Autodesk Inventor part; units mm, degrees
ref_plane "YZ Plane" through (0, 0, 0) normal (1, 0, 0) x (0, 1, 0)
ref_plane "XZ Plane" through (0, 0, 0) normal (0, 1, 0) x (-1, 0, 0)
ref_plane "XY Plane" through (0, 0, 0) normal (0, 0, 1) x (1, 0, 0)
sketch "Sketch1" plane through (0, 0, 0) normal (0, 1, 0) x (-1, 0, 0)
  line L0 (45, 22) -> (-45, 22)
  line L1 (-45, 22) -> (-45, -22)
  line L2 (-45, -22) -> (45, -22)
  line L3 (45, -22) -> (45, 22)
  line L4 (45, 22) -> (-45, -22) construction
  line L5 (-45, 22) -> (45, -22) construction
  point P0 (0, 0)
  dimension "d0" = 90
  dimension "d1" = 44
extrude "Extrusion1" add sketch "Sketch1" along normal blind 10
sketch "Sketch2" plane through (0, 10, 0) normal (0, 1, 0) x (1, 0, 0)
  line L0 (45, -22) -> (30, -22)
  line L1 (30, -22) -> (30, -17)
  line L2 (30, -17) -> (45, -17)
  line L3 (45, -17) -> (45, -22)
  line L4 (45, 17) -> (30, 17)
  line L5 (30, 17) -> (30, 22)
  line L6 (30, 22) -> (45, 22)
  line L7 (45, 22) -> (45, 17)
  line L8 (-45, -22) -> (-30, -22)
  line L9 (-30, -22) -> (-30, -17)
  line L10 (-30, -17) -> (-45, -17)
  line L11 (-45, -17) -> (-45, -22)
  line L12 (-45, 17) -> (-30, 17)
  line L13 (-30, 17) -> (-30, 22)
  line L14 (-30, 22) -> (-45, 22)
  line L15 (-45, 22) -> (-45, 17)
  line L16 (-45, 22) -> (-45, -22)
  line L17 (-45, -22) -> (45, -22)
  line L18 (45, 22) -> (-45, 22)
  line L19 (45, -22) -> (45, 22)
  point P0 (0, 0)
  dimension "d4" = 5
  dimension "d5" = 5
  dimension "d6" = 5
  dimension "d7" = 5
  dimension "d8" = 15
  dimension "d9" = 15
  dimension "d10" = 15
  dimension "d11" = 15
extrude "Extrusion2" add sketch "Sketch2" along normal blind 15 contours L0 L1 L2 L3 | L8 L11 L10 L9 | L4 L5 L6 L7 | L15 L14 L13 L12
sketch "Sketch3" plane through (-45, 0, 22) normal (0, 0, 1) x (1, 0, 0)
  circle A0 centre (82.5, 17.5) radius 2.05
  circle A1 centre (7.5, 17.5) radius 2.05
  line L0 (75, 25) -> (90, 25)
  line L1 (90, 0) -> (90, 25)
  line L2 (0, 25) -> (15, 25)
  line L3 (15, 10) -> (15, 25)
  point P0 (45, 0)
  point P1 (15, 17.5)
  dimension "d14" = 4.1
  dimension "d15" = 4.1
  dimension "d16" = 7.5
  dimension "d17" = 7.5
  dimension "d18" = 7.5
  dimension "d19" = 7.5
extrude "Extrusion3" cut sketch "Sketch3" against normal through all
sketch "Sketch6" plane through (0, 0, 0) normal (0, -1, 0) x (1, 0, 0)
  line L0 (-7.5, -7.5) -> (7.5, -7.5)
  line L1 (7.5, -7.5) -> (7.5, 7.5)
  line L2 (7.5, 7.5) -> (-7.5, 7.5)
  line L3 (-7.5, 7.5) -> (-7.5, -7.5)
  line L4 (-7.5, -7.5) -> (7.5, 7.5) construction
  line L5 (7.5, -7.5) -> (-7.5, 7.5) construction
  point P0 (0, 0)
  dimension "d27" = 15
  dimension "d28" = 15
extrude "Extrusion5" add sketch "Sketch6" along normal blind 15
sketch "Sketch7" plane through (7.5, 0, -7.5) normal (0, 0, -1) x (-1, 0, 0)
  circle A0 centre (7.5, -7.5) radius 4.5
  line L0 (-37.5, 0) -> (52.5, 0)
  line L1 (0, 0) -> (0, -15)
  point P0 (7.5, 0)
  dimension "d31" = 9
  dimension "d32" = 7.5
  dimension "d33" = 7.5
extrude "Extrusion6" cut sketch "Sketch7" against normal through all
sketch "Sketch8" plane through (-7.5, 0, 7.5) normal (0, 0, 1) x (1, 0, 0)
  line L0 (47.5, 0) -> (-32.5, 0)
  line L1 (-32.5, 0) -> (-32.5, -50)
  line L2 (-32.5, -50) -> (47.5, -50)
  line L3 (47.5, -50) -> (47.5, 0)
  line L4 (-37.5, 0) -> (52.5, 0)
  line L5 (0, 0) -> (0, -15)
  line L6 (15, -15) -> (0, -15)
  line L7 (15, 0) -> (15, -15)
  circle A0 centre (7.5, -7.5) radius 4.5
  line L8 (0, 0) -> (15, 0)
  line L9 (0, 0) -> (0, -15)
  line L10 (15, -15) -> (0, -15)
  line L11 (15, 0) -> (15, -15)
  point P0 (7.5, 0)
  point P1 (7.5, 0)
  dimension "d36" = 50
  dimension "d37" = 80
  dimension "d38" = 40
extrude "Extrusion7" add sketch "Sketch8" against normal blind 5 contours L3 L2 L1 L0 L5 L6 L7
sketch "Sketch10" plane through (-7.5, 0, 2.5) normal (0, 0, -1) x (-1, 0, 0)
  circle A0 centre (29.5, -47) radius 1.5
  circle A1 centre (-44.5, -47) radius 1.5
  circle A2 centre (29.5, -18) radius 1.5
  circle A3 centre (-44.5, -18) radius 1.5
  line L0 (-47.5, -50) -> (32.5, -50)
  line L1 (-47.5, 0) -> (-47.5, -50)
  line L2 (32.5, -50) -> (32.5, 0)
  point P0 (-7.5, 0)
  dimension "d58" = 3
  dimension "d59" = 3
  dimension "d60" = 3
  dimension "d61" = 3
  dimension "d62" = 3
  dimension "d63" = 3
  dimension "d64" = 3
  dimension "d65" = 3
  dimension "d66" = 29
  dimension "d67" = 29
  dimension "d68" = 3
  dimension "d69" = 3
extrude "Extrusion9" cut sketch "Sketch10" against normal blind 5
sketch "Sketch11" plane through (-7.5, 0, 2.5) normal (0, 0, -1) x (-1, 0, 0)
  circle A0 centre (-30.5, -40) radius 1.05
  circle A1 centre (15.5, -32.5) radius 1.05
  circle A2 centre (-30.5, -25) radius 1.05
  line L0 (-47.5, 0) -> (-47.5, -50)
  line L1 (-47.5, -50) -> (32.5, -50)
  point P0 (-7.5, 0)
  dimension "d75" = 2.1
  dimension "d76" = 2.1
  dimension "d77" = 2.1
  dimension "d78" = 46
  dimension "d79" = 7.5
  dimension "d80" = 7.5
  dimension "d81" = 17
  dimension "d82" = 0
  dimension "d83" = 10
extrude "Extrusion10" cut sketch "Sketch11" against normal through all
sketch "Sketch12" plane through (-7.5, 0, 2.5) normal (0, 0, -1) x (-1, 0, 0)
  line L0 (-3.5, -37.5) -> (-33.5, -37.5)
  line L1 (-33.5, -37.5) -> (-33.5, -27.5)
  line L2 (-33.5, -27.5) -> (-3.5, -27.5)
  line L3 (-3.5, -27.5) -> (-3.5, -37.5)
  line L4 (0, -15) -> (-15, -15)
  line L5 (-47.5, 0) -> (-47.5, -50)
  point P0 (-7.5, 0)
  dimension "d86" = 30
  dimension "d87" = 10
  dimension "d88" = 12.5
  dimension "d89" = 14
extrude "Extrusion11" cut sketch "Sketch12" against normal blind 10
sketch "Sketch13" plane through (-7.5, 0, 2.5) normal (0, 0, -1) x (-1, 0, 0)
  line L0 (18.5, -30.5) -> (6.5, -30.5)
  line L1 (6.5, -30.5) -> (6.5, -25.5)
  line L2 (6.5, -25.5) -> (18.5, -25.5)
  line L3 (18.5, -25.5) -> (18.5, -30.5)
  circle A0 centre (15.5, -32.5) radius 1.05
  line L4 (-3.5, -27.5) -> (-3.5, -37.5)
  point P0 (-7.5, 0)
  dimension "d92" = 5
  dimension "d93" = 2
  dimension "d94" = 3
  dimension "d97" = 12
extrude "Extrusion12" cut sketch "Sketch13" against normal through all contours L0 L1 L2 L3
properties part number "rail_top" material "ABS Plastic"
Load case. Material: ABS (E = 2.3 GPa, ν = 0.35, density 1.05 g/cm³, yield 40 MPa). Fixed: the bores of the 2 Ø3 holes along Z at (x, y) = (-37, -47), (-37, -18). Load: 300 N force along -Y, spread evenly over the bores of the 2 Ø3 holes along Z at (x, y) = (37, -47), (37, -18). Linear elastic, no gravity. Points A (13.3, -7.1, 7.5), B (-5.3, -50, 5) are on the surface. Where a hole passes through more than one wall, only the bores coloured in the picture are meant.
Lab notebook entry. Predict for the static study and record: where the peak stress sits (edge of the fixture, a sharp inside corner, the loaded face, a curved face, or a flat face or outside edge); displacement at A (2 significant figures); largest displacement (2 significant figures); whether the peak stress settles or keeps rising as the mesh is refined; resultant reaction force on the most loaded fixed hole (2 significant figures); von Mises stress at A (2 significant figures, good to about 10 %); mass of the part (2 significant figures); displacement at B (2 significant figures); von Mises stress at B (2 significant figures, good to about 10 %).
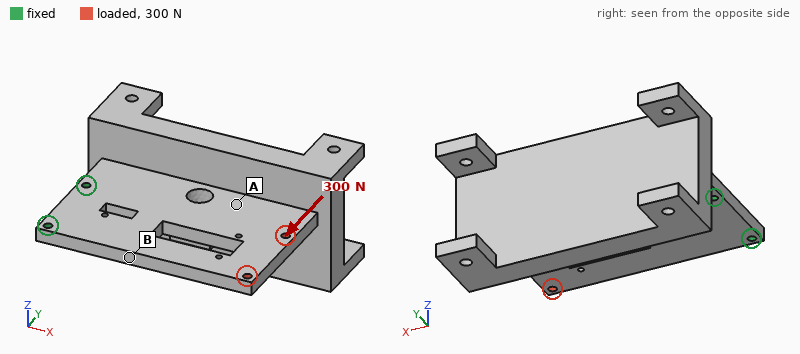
edge of the fixture
0.67 mm
1.3 mm
keeps rising
790 N
3.5 MPa
66 g
0.38 mm
7.5 MPa
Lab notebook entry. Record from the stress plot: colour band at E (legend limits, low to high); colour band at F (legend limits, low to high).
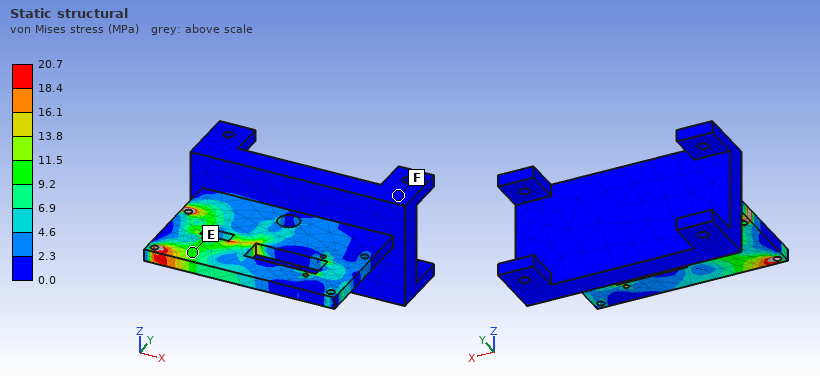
9.2 to 11.5 MPa
0.0 to 2.3 MPa
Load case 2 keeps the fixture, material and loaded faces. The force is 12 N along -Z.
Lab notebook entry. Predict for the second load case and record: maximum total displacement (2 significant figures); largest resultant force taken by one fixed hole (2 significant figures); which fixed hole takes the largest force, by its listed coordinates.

1.3 mm
9.0 N
(-37, -18)
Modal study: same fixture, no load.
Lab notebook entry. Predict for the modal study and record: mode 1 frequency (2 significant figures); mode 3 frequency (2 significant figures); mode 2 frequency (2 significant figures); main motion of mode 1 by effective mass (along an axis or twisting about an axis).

93 Hz
490 Hz
260 Hz
along Z
